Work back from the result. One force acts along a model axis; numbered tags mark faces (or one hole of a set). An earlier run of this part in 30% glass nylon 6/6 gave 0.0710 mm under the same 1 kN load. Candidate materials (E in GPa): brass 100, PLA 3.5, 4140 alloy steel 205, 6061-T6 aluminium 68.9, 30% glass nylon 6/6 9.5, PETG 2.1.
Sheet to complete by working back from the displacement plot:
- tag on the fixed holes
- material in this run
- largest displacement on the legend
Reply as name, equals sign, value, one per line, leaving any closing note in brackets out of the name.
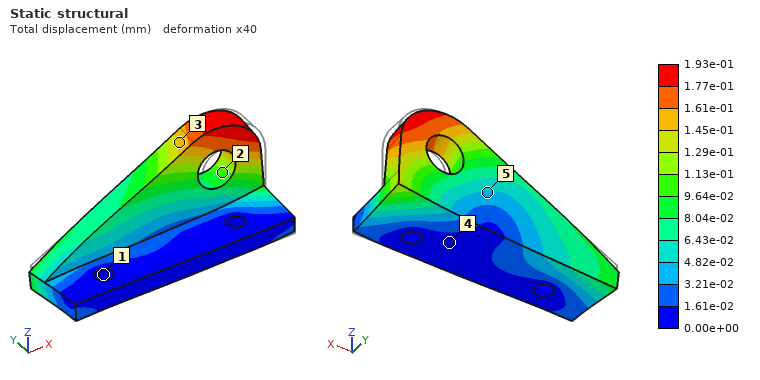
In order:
tag on the fixed holes = 1
material in this run = PLA
largest displacement on the legend = 1.93e-01 mm
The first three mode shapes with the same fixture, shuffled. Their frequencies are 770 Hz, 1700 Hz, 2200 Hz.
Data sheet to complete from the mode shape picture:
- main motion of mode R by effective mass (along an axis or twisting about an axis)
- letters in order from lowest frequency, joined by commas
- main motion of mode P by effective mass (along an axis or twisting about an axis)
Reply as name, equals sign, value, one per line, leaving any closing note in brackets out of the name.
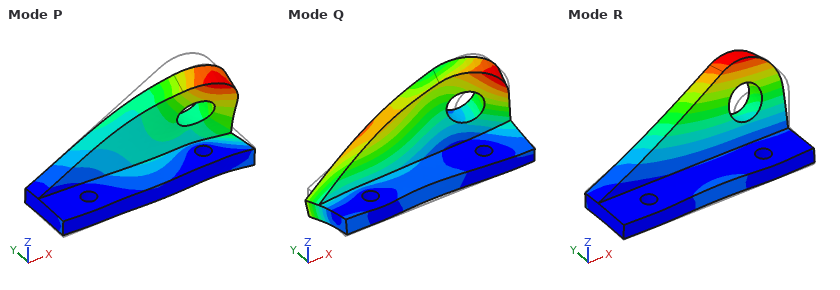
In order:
main motion of mode R by effective mass = along Y
letters in order from lowest frequency, joined by commas = R, Q, P
main motion of mode P by effective mass = along Z
